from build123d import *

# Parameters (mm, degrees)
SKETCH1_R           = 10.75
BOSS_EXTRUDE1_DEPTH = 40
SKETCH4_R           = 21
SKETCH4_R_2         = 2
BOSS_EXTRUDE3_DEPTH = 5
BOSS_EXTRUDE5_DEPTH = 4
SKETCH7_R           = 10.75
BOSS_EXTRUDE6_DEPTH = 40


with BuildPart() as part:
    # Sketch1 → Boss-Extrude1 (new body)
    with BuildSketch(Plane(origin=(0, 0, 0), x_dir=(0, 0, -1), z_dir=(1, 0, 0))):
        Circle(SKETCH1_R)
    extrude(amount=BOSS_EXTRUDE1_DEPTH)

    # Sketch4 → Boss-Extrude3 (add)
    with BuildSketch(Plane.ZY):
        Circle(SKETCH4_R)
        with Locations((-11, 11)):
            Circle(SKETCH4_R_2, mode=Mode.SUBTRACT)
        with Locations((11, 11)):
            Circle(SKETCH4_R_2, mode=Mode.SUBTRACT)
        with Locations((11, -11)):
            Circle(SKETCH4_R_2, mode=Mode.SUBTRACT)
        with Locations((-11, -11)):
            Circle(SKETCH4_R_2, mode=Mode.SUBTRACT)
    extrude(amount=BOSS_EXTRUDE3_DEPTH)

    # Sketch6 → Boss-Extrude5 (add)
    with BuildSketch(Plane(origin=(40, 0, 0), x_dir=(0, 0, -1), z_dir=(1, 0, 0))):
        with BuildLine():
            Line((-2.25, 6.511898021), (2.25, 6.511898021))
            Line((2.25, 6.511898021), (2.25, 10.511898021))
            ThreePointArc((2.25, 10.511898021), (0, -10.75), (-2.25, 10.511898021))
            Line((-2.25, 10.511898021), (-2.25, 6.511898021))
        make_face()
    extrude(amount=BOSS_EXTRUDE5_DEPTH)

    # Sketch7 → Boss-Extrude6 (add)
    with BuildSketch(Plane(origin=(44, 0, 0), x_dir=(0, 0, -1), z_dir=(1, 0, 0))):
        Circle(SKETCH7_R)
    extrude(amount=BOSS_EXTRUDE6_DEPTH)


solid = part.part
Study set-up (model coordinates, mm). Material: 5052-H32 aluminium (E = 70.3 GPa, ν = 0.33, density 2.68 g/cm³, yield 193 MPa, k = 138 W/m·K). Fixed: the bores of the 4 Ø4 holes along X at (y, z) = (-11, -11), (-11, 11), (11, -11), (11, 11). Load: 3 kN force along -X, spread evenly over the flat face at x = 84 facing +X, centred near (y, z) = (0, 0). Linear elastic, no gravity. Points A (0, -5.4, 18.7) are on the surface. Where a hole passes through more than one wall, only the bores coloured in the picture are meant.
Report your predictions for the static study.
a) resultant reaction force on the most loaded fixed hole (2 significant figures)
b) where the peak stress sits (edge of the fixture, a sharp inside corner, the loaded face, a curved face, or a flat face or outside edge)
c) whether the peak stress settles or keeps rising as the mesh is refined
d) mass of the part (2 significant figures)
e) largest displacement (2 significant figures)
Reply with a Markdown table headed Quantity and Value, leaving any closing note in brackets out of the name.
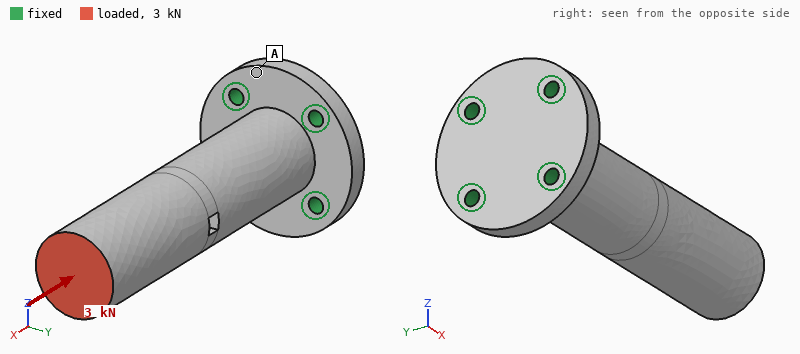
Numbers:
| Quantity | Value |
|---|---|
| resultant reaction force on the most loaded fixed hole | 780 N |
| where the peak stress sits | edge of the fixture |
| whether the peak stress settles or keeps rising as the mesh is refined | keeps rising |
| mass of the part | 99 g |
| largest displacement | 15 µm |
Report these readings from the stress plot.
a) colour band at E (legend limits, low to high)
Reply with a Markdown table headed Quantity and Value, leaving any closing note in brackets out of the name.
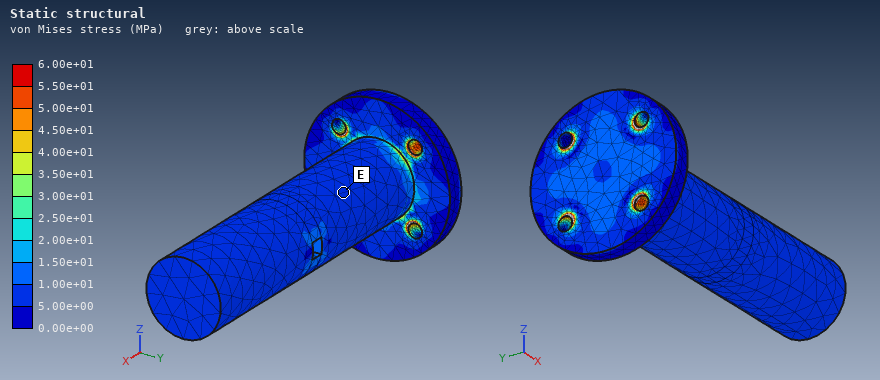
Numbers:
| Quantity | Value |
|---|---|
| colour band at E | 5.00e+00 to 1.00e+01 MPa |
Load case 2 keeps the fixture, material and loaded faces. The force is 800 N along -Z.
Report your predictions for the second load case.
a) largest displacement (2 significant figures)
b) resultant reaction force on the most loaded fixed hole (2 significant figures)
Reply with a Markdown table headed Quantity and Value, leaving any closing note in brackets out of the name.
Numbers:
| Quantity | Value |
|---|---|
| largest displacement | 0.33 mm |
| resultant reaction force on the most loaded fixed hole | 1.7 kN |
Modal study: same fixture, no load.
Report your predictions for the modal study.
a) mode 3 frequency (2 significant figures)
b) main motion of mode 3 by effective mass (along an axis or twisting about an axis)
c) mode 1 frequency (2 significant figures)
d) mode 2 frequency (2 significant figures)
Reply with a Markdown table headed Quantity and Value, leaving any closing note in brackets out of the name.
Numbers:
| Quantity | Value |
|---|---|
| mode 3 frequency | 8900 Hz |
| main motion of mode 3 by effective mass | twisting about X |
| mode 1 frequency | 1600 Hz |
| mode 2 frequency | 1600 Hz |
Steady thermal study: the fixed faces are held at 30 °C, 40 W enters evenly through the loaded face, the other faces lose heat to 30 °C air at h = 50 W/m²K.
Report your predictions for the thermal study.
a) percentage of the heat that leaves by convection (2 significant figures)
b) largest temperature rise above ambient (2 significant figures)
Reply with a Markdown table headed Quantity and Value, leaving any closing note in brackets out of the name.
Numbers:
| Quantity | Value |
|---|---|
| percentage of the heat that leaves by convection | 24 % |
| largest temperature rise above ambient | 63 K |
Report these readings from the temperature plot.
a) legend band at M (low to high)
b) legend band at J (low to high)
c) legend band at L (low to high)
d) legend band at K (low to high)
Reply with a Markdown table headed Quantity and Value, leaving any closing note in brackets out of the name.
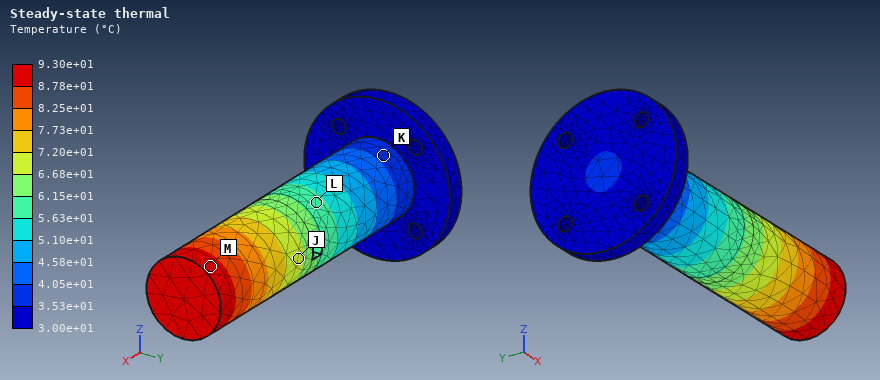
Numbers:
| Quantity | Value |
|---|---|
| legend band at M | 8.78e+01 to 9.30e+01 °C |
| legend band at J | 6.68e+01 to 7.20e+01 °C |
| legend band at L | 5.63e+01 to 6.15e+01 °C |
| legend band at K | 3.53e+01 to 4.05e+01 °C |
